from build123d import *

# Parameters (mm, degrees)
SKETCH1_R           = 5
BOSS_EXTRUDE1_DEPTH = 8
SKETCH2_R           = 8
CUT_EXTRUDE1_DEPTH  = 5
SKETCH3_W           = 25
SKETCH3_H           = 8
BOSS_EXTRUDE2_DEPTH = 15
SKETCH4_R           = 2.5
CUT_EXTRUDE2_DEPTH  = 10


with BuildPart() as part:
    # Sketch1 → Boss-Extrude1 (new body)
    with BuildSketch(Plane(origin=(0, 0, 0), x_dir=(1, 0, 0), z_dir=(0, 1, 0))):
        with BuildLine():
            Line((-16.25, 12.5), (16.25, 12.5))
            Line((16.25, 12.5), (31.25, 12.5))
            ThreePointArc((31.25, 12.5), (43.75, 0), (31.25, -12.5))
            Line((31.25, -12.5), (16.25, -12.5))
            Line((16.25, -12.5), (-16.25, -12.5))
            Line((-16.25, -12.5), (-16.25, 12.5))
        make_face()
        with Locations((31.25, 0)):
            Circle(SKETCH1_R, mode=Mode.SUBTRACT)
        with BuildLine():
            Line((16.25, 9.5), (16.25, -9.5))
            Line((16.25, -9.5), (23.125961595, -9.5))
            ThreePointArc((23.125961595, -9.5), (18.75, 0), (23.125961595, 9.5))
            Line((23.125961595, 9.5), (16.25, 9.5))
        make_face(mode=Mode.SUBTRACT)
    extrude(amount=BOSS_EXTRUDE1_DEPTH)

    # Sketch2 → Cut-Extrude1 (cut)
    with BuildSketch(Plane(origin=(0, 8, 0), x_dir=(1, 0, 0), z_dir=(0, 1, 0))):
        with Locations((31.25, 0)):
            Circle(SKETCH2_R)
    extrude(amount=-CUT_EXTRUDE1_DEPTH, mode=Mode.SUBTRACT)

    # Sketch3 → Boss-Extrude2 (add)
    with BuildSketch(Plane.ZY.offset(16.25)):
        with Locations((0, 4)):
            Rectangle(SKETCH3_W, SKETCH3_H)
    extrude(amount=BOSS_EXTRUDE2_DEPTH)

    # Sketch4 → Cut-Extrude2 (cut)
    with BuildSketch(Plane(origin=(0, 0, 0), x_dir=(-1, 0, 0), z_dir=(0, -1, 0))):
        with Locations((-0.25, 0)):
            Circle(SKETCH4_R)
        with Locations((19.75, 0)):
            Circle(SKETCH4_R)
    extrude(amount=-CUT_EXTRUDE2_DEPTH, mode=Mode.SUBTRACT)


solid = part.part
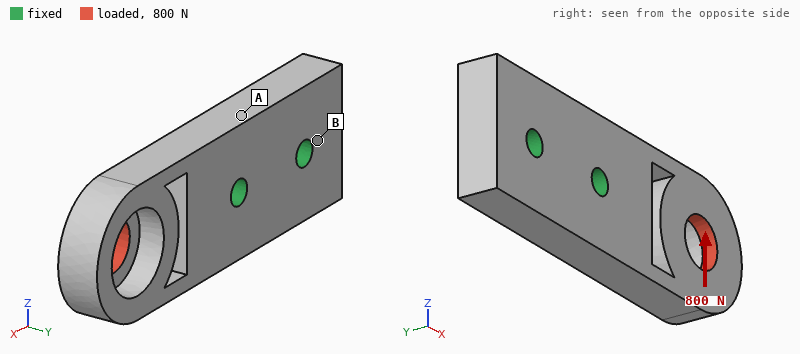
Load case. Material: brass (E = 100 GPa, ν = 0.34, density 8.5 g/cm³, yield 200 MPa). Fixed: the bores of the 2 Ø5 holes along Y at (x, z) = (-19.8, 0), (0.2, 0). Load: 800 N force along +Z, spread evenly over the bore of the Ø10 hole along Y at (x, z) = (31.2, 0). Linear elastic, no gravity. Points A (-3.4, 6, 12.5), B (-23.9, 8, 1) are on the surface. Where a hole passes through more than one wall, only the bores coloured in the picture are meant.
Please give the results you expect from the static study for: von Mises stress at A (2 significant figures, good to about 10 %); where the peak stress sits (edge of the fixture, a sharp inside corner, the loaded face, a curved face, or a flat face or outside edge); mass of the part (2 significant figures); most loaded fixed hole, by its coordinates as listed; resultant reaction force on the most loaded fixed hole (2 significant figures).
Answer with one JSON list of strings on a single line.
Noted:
["24 MPa", "a flat face or outside edge", "100 g", "(0.2, 0)", "1.6 kN"]
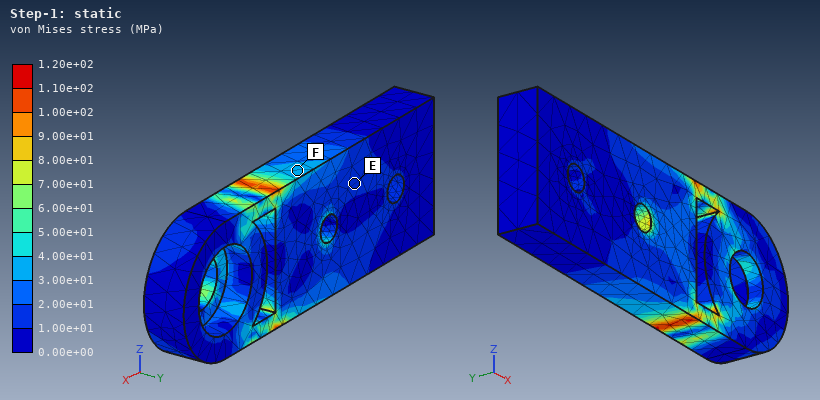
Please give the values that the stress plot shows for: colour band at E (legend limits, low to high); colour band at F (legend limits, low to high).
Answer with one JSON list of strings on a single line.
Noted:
["1.00e+01 to 2.00e+01 MPa", "3.00e+01 to 4.00e+01 MPa"]
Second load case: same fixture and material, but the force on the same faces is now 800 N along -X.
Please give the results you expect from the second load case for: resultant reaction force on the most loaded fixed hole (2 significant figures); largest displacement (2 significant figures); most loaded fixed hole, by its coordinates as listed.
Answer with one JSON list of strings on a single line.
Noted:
["610 N", "39 µm", "(0.2, 0)"]
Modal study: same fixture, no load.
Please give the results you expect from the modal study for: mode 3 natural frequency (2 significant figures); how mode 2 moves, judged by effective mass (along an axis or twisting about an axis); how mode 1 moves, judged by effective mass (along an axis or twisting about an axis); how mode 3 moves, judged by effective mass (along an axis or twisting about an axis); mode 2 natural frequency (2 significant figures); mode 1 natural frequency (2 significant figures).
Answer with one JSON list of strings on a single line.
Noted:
["6200 Hz", "along Z", "along Y", "twisting about X", "4000 Hz", "2300 Hz"]
